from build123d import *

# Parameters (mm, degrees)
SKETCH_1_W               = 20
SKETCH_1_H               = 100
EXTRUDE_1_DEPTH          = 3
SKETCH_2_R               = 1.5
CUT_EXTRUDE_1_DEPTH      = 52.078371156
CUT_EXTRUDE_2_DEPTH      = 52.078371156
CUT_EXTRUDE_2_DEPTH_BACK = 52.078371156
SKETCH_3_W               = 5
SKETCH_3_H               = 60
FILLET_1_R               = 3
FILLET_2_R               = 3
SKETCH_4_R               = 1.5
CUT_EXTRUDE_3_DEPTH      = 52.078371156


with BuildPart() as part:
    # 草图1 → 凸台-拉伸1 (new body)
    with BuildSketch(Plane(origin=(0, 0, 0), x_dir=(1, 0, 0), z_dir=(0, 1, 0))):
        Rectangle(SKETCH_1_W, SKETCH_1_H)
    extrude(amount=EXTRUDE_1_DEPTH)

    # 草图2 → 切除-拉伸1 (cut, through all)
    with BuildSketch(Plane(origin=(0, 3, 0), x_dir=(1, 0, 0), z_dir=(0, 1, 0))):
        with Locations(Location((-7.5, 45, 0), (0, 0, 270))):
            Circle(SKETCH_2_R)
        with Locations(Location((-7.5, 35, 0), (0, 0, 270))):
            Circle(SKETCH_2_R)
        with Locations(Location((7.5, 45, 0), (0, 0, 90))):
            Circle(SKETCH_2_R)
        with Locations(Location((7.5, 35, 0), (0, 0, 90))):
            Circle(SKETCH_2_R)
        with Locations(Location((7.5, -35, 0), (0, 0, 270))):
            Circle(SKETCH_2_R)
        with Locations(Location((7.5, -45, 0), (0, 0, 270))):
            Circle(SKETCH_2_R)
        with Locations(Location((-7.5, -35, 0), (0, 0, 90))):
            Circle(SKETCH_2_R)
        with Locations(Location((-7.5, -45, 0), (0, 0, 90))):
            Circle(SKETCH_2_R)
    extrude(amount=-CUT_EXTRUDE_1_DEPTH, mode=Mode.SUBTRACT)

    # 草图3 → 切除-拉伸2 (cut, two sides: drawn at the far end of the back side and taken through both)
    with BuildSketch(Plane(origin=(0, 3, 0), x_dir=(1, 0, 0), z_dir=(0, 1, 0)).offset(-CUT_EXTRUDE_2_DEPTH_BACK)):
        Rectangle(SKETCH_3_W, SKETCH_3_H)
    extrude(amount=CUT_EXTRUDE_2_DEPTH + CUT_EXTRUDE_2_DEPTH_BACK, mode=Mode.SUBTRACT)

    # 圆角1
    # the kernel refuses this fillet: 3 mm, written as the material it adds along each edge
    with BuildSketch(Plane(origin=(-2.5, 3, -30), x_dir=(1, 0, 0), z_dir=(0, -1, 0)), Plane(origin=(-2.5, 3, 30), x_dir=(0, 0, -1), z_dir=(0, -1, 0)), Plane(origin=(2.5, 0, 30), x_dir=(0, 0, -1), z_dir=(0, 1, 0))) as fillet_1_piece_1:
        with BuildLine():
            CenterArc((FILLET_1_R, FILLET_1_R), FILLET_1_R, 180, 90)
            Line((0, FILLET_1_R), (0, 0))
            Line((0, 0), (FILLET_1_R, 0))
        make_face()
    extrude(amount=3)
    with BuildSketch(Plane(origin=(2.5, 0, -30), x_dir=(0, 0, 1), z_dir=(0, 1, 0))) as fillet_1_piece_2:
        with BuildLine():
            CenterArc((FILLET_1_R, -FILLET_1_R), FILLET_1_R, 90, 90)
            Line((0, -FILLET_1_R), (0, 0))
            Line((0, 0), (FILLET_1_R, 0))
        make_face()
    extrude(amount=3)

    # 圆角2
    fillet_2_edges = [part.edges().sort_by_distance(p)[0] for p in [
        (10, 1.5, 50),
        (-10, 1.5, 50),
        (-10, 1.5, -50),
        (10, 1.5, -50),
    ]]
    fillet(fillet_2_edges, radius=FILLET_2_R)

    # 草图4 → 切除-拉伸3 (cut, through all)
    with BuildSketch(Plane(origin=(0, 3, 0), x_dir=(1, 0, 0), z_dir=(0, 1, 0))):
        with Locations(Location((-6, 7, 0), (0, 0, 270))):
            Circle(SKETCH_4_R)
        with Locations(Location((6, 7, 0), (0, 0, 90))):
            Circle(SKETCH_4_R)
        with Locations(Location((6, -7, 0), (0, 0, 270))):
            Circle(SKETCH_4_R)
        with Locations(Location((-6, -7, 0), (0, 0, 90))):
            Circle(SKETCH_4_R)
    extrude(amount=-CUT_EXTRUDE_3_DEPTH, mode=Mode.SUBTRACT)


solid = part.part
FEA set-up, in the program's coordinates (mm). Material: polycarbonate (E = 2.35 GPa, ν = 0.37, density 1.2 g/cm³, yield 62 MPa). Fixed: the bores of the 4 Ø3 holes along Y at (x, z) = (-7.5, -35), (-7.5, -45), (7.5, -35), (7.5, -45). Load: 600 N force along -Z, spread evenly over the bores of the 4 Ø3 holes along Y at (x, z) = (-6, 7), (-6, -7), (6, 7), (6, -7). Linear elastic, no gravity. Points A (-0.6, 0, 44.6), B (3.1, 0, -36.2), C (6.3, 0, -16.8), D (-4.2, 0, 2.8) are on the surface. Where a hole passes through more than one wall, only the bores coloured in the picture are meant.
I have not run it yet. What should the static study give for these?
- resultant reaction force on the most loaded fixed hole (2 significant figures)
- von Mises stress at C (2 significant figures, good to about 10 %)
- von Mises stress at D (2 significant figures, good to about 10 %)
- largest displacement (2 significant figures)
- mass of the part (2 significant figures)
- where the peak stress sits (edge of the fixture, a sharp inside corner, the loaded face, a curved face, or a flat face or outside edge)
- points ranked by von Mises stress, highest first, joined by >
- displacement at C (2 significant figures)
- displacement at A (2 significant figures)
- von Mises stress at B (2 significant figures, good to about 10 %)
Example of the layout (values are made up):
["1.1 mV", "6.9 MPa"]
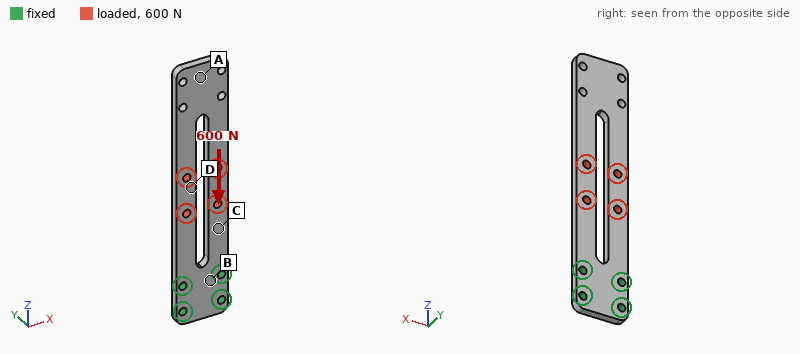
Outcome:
["270 N", "13 MPa", "6.8 MPa", "0.22 mm", "5.8 g", "the loaded face", "C > D > B > A", "0.10 mm", "0.21 mm", "3.6 MPa"]
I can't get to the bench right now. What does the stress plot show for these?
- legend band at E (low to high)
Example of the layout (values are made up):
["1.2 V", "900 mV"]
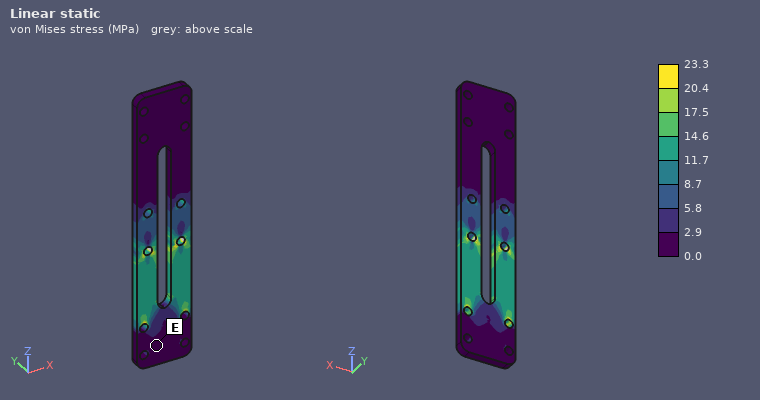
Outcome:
["0.0 to 2.9 MPa"]
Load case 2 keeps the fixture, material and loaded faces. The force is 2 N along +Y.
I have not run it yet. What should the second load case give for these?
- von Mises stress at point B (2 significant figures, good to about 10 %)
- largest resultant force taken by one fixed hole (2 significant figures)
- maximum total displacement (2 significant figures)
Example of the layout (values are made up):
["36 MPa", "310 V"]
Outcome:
["0.70 MPa", "1.8 N", "1.1 mm"]
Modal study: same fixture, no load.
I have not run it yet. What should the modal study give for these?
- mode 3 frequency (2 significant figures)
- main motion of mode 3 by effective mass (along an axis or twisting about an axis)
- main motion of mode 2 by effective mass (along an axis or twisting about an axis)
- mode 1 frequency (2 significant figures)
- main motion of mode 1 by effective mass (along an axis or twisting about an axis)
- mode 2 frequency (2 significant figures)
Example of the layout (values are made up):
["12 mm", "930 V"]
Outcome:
["580 Hz", "twisting about Z", "along X", "88 Hz", "along Y", "400 Hz"]
